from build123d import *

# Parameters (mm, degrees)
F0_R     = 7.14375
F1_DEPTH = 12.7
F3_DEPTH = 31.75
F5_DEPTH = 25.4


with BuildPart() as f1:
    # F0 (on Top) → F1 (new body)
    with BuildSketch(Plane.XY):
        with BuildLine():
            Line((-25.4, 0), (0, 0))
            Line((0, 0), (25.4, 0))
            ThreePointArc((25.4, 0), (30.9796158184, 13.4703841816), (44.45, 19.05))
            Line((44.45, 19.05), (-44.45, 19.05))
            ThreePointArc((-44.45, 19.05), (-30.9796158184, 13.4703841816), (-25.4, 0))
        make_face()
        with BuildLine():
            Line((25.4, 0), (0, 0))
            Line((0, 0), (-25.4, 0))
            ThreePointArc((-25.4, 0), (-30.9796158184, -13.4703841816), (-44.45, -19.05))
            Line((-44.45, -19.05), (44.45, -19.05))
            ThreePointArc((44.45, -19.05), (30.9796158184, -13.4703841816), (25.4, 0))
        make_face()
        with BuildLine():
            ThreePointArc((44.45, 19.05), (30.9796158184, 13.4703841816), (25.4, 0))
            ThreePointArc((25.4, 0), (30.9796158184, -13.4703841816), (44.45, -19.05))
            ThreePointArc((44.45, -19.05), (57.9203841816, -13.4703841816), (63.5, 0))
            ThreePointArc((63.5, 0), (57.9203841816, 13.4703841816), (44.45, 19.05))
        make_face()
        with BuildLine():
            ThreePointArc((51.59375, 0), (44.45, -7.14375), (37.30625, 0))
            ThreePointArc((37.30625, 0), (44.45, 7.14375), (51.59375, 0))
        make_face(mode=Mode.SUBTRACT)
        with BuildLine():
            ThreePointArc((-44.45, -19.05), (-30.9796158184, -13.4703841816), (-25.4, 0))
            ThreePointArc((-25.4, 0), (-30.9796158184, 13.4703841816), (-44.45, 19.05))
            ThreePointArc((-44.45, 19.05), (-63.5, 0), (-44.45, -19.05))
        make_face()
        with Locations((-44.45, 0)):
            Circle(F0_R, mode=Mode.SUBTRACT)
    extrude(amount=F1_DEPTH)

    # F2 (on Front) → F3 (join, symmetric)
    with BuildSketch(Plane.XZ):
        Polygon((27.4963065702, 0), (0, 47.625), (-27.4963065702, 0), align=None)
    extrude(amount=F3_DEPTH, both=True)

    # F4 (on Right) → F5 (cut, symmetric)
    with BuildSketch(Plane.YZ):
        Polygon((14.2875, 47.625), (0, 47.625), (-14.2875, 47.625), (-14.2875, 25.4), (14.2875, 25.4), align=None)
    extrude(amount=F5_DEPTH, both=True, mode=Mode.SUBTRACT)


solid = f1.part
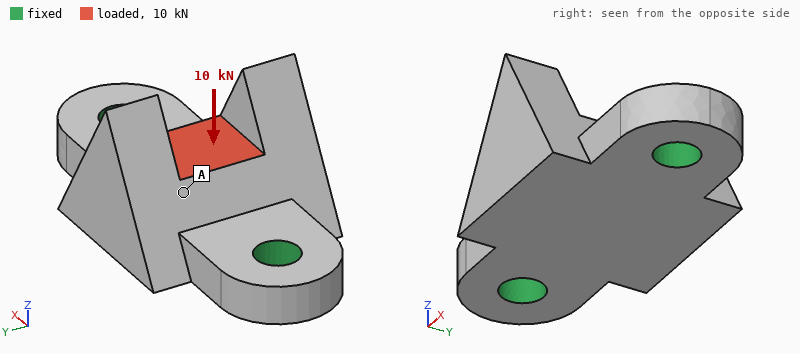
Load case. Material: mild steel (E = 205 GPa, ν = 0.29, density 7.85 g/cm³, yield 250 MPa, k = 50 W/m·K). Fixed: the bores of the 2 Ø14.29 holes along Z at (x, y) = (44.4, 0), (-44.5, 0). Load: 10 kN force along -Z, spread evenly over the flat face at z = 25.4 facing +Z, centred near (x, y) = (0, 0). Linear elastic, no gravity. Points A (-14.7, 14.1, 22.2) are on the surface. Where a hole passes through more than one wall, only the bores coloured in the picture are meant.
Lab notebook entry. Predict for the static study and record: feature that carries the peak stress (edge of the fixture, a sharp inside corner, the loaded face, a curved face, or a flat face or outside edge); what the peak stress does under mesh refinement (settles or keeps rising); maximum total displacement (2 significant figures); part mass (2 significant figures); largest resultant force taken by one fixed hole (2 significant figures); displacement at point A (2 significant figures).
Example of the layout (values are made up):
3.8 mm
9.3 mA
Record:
edge of the fixture
keeps rising
11 µm
830 g
5.3 kN
10 µm
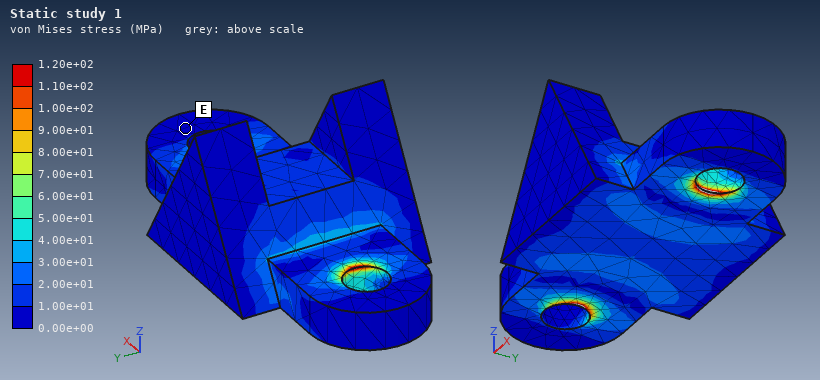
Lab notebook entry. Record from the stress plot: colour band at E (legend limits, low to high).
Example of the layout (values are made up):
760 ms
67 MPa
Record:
0.00e+00 to 1.00e+01 MPa
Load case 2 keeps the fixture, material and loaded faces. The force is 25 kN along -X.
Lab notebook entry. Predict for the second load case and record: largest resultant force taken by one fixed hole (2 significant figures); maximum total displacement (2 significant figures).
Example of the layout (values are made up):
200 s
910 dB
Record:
15 kN
24 µm
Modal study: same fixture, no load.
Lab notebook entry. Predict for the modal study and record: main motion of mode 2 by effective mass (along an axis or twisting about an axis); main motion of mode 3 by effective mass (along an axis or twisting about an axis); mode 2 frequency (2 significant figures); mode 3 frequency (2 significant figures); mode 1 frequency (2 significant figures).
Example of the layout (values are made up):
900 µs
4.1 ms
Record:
along Z
along Y
6200 Hz
10 kHz
3800 Hz
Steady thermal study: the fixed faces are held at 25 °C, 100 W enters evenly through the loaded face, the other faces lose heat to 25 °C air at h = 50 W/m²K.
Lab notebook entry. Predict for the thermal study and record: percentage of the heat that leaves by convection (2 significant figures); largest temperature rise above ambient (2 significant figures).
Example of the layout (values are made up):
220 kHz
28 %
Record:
26 %
72 K
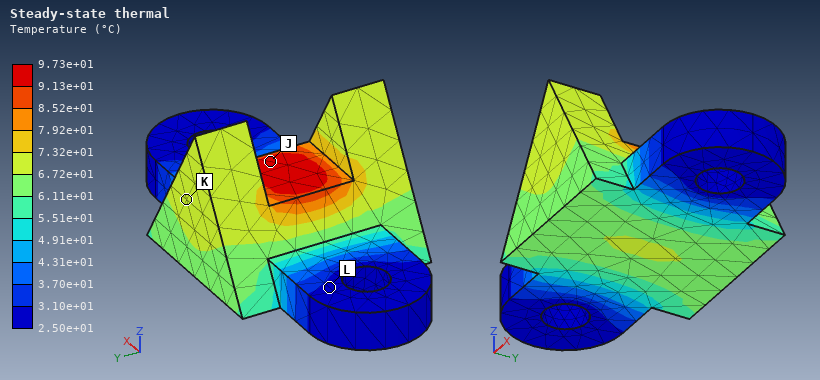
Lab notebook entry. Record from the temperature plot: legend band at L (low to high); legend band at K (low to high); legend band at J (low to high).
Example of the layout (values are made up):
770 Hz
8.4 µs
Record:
2.50e+01 to 3.10e+01 °C
6.72e+01 to 7.32e+01 °C
9.13e+01 to 9.73e+01 °C
